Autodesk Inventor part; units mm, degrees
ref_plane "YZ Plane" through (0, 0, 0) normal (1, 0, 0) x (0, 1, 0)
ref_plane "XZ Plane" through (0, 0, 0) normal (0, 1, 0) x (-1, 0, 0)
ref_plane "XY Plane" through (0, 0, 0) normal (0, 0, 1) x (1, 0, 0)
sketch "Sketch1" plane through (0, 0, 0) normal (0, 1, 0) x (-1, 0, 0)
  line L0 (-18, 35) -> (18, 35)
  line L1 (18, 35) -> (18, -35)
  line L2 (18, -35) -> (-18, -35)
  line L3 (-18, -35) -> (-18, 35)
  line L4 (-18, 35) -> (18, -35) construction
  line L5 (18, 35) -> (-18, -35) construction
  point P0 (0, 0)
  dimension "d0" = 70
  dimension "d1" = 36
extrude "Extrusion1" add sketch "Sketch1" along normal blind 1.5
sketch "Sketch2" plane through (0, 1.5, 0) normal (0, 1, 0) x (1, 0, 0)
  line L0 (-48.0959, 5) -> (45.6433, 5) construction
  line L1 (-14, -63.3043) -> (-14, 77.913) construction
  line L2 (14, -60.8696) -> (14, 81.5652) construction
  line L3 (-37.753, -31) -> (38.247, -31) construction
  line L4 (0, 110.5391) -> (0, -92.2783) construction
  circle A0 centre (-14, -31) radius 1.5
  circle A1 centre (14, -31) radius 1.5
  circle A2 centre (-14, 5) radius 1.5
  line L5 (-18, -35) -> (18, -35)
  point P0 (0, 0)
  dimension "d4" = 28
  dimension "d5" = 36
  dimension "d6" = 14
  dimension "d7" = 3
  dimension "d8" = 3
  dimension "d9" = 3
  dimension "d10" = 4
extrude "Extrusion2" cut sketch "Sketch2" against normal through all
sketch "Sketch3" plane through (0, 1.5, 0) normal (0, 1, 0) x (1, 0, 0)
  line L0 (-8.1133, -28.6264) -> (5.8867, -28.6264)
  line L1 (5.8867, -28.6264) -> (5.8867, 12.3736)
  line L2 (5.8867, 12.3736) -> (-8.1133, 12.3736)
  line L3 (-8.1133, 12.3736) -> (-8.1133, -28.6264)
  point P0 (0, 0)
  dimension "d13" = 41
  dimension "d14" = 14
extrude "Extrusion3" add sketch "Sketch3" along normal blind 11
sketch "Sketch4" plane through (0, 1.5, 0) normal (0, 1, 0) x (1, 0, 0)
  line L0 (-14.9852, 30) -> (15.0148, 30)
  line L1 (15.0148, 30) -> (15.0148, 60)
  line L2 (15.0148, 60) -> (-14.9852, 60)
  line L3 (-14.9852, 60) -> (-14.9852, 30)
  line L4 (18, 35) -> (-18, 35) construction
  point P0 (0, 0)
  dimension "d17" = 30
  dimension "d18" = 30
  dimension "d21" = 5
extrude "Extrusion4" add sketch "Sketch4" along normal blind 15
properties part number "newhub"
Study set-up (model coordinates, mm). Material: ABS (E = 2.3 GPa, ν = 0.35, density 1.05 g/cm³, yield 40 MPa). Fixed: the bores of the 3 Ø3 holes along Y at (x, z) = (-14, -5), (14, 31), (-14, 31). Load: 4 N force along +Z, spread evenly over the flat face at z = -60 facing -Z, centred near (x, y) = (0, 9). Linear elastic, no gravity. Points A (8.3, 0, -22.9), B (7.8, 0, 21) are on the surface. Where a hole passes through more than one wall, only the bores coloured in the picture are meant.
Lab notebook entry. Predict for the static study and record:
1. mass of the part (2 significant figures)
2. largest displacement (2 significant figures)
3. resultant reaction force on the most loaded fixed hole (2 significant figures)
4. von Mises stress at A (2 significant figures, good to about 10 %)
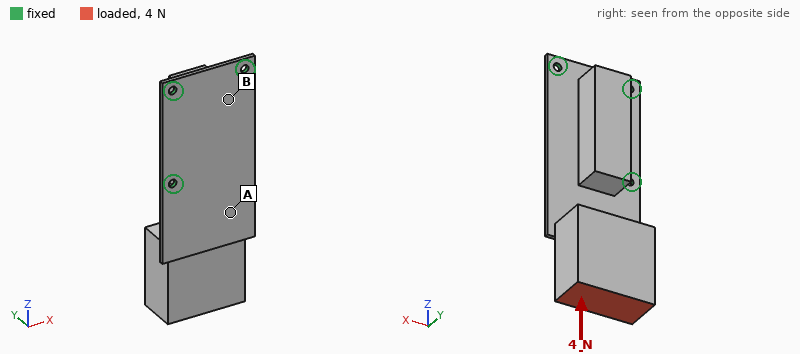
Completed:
25 g
1.1 mm
1.9 N
2.1 MPa
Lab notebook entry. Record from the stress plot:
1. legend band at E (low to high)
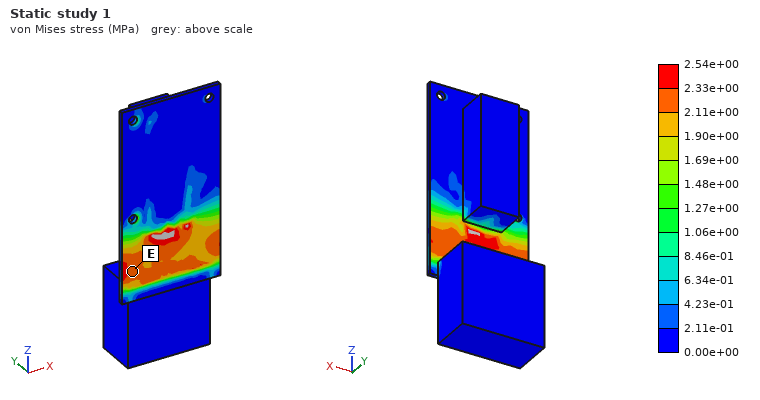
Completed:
2.11e+00 to 2.33e+00 MPa
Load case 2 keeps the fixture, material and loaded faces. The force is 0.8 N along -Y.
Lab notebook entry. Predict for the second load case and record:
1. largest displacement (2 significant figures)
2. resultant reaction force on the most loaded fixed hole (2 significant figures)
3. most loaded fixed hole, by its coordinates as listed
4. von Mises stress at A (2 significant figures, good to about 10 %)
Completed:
1.1 mm
2.1 N
(-14, -5)
1.9 MPa
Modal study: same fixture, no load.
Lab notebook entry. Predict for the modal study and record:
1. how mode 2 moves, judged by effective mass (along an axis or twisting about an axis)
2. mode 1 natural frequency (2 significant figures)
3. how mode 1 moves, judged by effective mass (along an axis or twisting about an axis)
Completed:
along X
52 Hz
along Y
